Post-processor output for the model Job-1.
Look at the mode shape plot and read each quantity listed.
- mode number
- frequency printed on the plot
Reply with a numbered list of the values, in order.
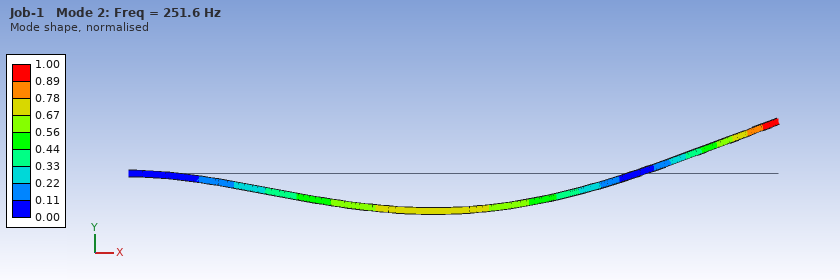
1. 2
2. 251.6 Hz
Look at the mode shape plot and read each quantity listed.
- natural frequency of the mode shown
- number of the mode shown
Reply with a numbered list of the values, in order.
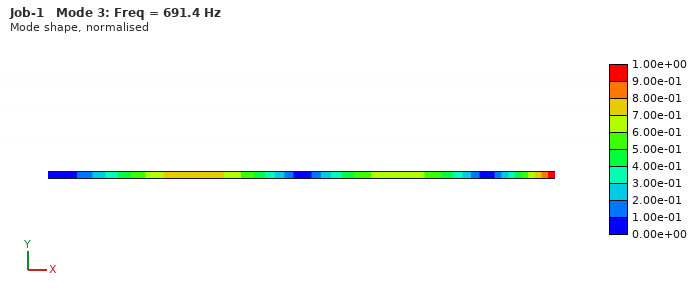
1. 691.4 Hz
2. 3
